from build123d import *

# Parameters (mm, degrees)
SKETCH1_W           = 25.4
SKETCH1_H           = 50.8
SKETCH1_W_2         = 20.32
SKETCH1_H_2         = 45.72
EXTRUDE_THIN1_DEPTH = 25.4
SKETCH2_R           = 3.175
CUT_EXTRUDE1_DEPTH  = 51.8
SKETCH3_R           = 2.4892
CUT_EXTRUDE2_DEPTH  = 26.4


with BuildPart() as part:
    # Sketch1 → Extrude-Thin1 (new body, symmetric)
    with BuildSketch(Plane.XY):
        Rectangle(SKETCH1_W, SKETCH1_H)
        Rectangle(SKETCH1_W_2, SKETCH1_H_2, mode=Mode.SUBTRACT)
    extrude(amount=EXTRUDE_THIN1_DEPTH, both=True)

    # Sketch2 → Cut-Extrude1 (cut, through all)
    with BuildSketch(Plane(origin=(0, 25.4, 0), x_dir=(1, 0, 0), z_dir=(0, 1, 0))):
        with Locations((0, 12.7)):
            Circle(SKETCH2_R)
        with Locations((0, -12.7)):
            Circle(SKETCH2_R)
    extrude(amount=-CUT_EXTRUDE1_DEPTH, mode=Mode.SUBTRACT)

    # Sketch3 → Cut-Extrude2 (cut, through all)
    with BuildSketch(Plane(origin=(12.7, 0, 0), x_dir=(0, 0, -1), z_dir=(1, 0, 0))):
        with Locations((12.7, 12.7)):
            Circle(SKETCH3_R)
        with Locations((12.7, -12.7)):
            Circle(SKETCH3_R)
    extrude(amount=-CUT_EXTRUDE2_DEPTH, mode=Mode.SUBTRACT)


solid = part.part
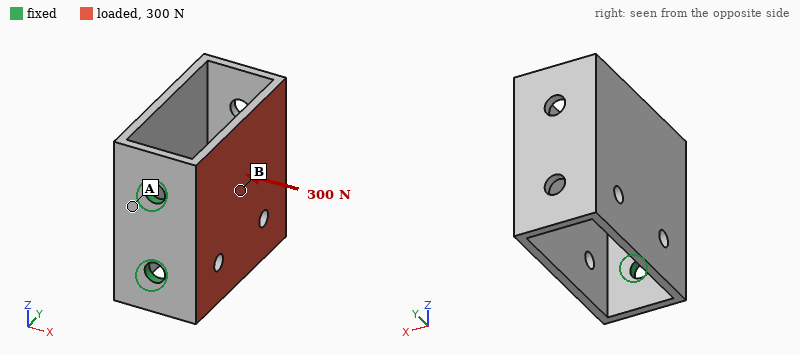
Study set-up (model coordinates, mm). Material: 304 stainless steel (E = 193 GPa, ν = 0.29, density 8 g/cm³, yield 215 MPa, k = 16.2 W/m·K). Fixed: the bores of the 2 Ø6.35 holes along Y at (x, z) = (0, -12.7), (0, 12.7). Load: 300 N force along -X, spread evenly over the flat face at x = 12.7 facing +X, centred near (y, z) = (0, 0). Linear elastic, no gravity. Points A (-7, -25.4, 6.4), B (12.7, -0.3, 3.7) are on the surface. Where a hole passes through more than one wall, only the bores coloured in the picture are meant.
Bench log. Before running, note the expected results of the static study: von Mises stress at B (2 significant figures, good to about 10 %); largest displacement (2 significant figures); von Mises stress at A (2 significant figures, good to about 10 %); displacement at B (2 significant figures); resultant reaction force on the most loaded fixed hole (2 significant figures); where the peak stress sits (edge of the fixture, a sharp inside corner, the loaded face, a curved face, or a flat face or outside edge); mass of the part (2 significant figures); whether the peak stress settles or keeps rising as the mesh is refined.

13 MPa
0.13 mm
39 MPa
0.079 mm
150 N
edge of the fixture
140 g
keeps rising
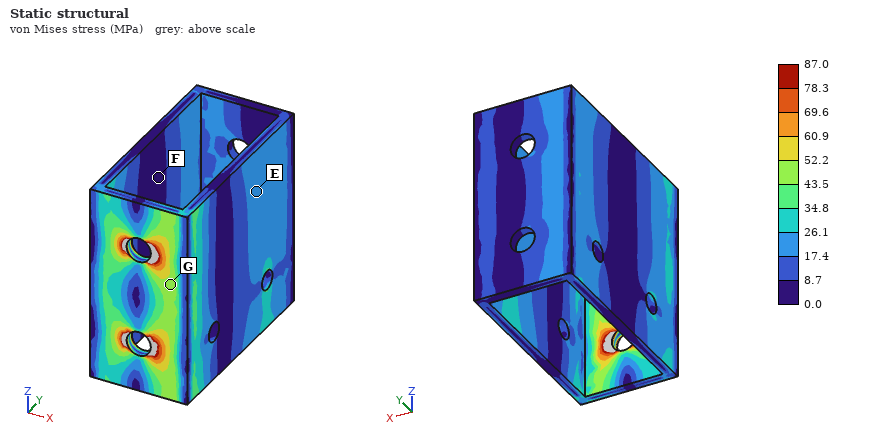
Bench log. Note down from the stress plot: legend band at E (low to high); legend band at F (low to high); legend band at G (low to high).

17.4 to 26.1 MPa
0.0 to 8.7 MPa
43.5 to 52.2 MPa
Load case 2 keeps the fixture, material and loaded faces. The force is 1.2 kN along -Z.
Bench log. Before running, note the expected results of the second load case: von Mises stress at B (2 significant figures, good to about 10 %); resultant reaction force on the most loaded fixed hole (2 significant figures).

37 MPa
1.2 kN
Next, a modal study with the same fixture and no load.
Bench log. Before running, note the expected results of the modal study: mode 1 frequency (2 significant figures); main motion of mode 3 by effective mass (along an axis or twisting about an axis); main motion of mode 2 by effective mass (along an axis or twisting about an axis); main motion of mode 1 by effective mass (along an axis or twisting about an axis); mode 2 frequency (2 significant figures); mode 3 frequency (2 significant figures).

710 Hz
twisting about Y
along Z
along X
2000 Hz
2400 Hz
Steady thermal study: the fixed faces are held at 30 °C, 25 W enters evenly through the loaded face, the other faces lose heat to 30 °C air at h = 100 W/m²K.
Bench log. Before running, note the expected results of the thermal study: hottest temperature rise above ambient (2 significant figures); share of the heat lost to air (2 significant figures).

60 K
83 %
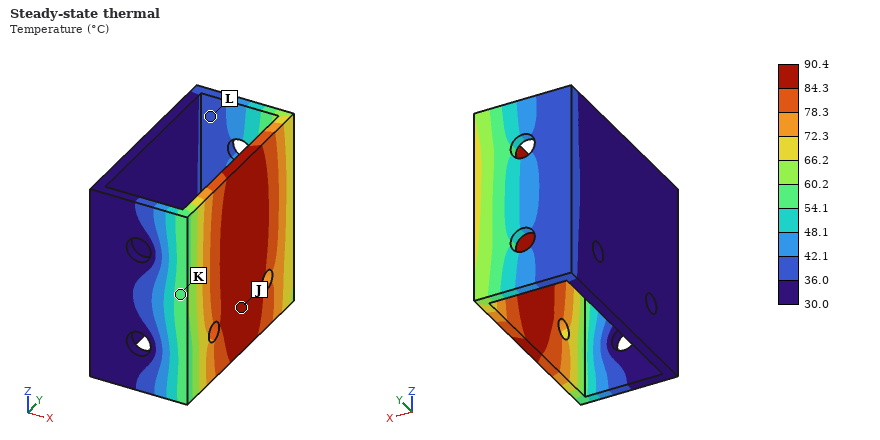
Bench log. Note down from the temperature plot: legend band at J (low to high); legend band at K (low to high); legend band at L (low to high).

84.3 to 90.4 °C
54.1 to 60.2 °C
36.0 to 42.1 °C
